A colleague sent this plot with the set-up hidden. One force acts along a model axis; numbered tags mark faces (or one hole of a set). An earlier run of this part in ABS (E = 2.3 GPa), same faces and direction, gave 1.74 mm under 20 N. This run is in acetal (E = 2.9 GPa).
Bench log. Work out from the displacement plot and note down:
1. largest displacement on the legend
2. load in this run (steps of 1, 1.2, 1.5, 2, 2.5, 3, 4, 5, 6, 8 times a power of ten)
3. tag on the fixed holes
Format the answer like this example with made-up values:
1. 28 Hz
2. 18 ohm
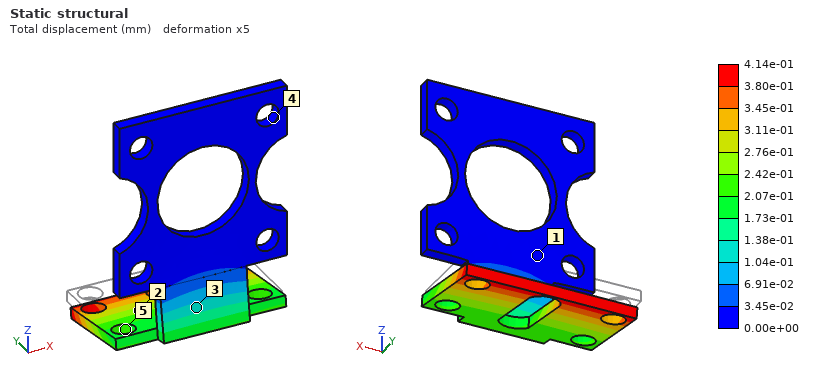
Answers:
1. 4.14e-01 mm
2. 6 N
3. 4
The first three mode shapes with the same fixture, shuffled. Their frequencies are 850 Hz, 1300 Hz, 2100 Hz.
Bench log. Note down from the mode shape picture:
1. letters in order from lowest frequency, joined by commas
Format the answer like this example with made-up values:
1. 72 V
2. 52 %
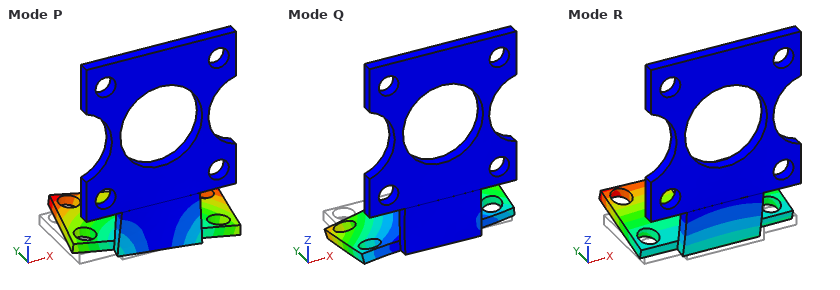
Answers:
1. R, P, Q
